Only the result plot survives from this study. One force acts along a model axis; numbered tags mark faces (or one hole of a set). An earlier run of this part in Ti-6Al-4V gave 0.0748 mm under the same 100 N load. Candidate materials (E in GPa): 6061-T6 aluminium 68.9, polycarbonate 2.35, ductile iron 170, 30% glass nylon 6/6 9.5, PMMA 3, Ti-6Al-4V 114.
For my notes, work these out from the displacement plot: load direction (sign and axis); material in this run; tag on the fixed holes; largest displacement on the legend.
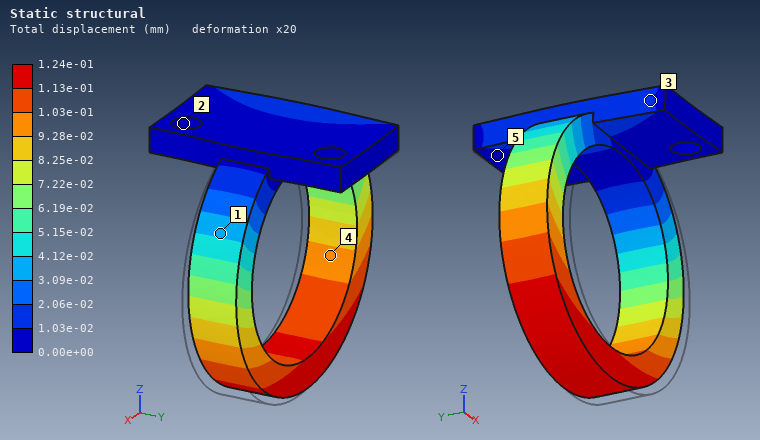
-X
6061-T6 aluminium
2
1.24e-01 mm
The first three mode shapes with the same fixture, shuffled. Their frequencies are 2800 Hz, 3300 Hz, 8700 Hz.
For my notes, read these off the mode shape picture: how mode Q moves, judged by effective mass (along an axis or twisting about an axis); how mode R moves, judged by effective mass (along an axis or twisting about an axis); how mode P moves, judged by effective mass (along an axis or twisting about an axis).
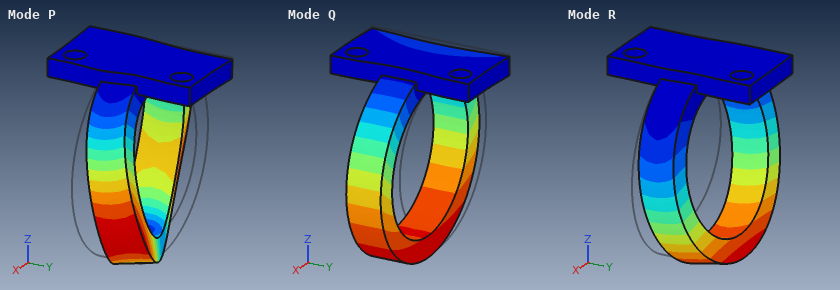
along X
along Y
twisting about Z
